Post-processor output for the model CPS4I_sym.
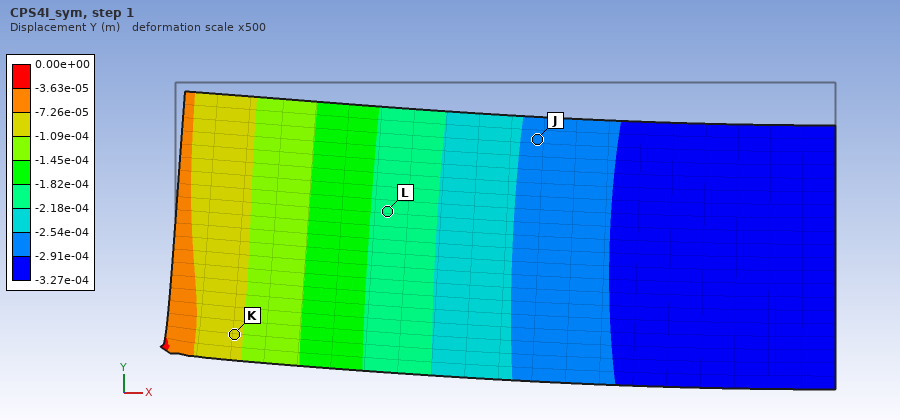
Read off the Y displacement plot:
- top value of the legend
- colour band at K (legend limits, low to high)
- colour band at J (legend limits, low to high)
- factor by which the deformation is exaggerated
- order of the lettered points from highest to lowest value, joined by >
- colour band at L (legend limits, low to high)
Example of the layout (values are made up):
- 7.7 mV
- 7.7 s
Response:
- 0.00e+00 m
- -1.09e-04 to -7.26e-05 m
- -2.91e-04 to -2.54e-04 m
- 500
- K > L > J
- -2.18e-04 to -1.82e-04 m
